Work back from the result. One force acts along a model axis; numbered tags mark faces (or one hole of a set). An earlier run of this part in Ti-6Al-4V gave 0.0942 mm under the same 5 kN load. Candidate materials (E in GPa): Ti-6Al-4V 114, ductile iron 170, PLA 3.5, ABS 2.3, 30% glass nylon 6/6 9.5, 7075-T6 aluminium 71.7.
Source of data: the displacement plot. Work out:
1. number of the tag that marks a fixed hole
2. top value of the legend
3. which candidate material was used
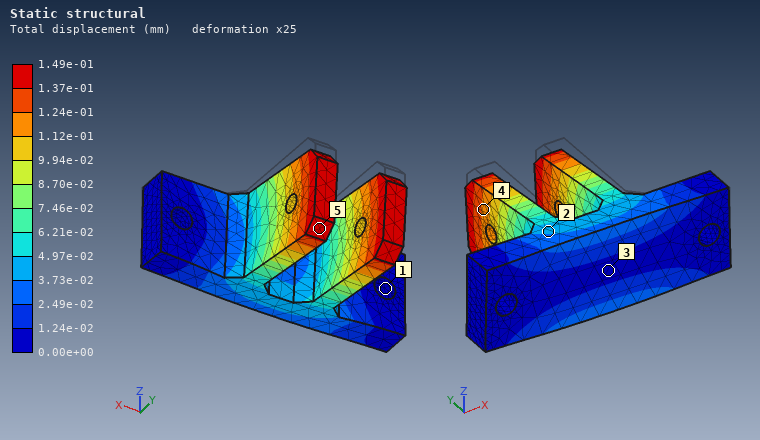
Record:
1
1.49e-01 mm
7075-T6 aluminium
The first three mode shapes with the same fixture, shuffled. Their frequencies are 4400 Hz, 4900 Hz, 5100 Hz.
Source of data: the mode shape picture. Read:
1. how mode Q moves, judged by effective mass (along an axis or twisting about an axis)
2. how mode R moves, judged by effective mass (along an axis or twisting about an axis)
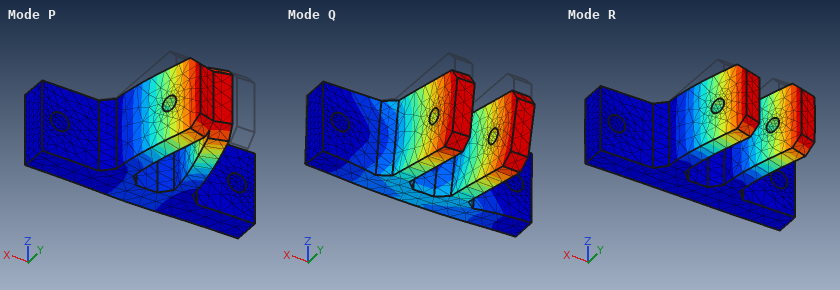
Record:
along Z
along X
